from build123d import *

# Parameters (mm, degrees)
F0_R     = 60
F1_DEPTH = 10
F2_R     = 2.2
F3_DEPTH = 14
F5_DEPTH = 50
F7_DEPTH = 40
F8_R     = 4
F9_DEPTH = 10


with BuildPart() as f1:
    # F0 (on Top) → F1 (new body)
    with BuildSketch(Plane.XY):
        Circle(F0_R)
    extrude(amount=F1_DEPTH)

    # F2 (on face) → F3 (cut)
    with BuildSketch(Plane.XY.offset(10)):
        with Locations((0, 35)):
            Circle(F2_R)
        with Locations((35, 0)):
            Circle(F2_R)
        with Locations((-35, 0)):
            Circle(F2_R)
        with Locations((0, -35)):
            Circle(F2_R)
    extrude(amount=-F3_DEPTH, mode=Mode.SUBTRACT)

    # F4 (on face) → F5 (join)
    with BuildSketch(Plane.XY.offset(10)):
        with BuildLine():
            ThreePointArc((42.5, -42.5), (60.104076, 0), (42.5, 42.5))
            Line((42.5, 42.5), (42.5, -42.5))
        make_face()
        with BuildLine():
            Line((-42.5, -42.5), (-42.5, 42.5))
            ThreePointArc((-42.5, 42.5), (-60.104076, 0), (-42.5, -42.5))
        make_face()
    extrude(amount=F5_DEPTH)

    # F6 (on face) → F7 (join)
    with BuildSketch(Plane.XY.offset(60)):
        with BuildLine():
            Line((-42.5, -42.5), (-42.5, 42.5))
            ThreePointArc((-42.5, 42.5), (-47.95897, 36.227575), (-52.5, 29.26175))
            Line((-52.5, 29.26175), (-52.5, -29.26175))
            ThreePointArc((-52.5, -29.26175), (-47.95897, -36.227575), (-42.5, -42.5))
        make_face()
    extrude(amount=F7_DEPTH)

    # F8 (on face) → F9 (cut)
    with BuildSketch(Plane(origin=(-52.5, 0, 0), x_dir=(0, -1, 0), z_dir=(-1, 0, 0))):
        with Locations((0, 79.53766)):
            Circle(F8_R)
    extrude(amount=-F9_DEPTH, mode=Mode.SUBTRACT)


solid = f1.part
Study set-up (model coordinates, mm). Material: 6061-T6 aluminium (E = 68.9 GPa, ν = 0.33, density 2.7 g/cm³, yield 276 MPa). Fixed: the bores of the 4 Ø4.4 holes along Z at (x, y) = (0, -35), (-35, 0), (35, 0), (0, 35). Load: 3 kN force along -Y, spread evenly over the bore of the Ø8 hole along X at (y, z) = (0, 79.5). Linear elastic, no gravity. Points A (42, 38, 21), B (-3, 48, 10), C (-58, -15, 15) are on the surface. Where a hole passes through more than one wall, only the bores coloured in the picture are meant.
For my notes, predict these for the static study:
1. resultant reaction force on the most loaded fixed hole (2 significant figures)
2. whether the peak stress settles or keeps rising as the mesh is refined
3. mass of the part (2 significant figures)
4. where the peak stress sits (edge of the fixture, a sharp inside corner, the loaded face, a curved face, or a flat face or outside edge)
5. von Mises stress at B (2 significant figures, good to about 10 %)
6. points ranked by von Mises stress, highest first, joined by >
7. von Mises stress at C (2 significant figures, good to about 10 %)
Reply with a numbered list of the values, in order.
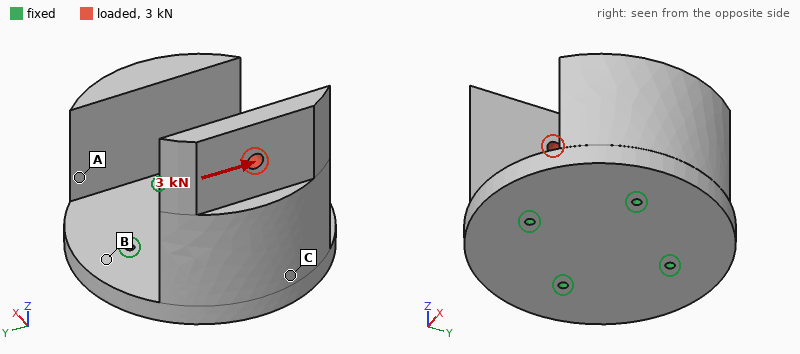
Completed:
1. 2.5 kN
2. keeps rising
3. 660 g
4. edge of the fixture
5. 38 MPa
6. B > C > A
7. 27 MPa
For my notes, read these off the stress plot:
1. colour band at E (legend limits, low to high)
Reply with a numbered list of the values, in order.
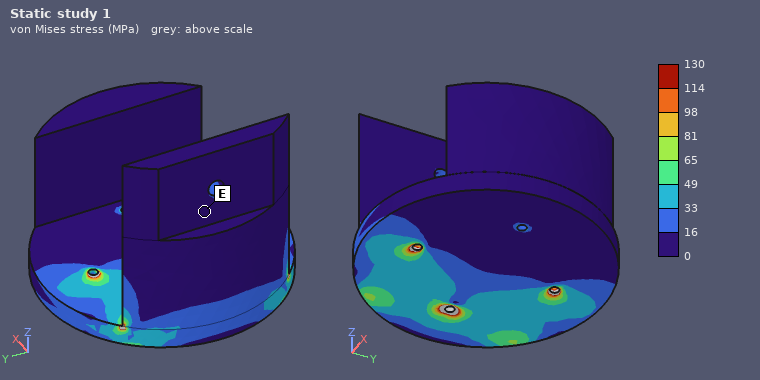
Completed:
1. 0 to 16 MPa
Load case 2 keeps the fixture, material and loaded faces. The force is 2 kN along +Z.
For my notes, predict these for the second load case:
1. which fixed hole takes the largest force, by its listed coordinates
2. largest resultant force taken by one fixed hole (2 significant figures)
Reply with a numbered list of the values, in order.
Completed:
1. (-35, 0)
2. 2.2 kN
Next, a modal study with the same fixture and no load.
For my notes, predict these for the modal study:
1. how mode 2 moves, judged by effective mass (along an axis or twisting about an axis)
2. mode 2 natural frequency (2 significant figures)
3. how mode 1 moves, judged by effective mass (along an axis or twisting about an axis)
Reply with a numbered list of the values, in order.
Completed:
1. along Y
2. 1400 Hz
3. along X
